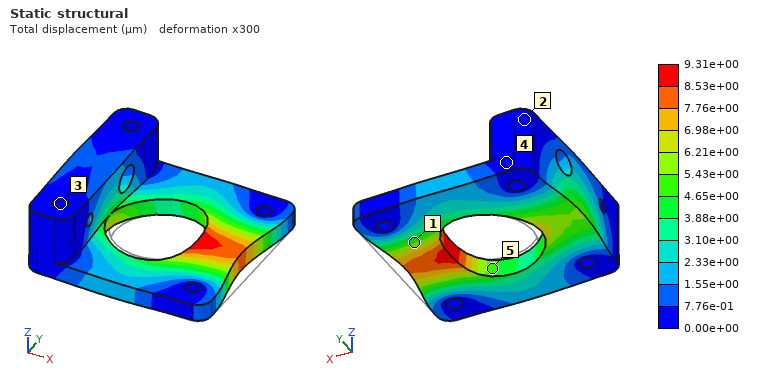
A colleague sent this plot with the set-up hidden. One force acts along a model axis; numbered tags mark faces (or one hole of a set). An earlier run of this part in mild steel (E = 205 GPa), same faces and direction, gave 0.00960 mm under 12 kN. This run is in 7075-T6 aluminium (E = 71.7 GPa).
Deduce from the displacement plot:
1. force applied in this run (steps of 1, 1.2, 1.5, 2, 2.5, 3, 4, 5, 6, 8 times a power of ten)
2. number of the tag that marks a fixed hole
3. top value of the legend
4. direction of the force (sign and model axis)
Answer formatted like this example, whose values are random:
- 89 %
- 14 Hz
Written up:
- 4 kN
- 3
- 9.31e+00 µm
- -X
